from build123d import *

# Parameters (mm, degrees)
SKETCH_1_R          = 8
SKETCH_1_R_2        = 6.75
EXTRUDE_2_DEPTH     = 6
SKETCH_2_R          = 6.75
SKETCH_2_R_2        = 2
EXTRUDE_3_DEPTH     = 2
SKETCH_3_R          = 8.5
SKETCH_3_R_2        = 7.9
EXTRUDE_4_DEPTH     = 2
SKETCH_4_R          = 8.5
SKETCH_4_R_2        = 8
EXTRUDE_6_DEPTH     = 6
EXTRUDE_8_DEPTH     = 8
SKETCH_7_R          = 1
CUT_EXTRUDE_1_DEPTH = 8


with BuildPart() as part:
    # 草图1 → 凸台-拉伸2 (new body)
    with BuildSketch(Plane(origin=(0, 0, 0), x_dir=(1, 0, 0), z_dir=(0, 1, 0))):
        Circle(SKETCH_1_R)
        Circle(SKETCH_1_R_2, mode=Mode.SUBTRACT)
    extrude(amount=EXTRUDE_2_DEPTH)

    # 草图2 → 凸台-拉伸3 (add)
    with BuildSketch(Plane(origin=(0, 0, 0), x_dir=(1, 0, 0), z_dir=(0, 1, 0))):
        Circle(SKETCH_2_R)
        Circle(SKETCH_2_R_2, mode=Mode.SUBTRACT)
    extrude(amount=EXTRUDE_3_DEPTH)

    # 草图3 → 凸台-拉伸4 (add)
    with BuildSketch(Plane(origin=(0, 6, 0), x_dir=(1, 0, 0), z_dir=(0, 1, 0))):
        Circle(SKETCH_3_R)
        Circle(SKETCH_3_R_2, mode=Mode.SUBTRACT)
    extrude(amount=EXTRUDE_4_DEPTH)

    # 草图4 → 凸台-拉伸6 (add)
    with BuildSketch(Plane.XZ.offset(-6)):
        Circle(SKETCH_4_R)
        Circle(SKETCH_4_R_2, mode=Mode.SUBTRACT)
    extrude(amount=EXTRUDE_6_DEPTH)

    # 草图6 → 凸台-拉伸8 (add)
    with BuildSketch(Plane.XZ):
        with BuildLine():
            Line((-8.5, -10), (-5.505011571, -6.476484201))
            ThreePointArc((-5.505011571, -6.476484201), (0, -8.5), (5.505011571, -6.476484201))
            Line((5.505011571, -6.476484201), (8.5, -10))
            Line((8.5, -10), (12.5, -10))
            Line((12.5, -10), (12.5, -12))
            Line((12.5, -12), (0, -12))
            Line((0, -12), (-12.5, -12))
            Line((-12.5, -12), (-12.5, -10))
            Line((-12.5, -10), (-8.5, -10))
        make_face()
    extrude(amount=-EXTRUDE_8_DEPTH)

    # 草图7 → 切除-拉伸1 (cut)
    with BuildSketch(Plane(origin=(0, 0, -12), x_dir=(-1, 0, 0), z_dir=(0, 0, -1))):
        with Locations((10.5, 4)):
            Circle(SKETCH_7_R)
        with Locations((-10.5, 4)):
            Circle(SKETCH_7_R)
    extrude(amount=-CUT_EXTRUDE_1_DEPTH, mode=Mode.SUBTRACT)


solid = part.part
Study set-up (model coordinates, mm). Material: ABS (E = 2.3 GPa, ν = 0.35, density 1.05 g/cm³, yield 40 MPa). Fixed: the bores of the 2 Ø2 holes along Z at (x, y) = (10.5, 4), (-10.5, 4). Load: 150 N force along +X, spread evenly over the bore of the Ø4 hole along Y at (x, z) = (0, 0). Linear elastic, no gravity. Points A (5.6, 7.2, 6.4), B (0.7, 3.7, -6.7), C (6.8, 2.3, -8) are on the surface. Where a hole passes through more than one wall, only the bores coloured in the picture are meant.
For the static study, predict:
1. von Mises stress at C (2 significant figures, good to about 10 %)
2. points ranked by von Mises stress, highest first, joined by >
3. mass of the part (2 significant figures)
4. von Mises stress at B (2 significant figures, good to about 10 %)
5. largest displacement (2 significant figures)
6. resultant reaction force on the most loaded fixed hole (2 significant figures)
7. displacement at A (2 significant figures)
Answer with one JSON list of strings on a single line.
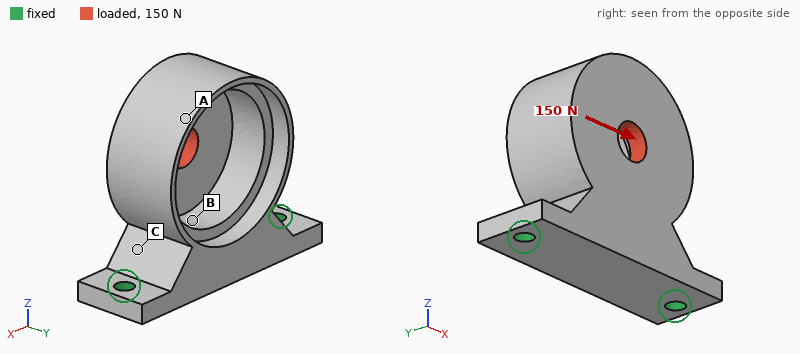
["18 MPa", "C > B > A", "1.6 g", "8.3 MPa", "0.37 mm", "120 N", "0.35 mm"]
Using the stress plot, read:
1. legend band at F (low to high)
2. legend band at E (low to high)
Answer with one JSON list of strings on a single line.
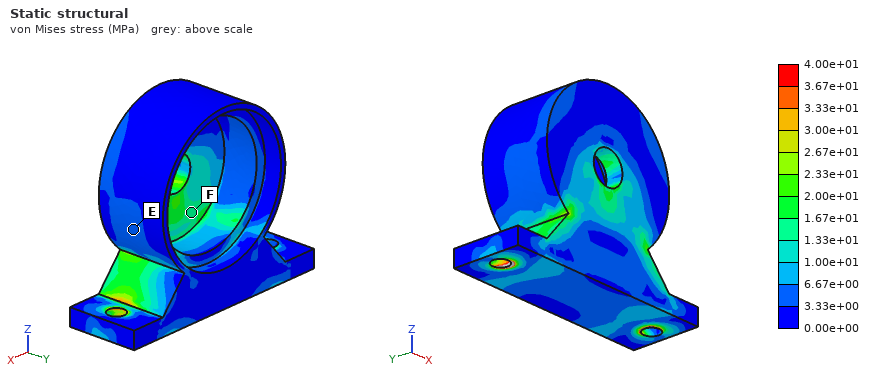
["1.33e+01 to 1.67e+01 MPa", "3.33e+00 to 6.67e+00 MPa"]
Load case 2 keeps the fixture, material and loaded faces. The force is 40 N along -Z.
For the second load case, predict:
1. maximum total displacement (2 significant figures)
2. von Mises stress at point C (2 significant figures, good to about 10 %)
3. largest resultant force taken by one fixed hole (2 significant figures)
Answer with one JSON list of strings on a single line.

["0.20 mm", "4.2 MPa", "25 N"]
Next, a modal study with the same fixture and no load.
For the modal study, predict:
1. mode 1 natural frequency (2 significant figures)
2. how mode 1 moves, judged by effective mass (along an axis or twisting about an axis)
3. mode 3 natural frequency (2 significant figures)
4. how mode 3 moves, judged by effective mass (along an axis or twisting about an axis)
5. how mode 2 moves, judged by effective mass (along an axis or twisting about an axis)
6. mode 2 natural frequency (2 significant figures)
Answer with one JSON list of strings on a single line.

["1400 Hz", "along Y", "5600 Hz", "along Z", "along X", "3600 Hz"]
